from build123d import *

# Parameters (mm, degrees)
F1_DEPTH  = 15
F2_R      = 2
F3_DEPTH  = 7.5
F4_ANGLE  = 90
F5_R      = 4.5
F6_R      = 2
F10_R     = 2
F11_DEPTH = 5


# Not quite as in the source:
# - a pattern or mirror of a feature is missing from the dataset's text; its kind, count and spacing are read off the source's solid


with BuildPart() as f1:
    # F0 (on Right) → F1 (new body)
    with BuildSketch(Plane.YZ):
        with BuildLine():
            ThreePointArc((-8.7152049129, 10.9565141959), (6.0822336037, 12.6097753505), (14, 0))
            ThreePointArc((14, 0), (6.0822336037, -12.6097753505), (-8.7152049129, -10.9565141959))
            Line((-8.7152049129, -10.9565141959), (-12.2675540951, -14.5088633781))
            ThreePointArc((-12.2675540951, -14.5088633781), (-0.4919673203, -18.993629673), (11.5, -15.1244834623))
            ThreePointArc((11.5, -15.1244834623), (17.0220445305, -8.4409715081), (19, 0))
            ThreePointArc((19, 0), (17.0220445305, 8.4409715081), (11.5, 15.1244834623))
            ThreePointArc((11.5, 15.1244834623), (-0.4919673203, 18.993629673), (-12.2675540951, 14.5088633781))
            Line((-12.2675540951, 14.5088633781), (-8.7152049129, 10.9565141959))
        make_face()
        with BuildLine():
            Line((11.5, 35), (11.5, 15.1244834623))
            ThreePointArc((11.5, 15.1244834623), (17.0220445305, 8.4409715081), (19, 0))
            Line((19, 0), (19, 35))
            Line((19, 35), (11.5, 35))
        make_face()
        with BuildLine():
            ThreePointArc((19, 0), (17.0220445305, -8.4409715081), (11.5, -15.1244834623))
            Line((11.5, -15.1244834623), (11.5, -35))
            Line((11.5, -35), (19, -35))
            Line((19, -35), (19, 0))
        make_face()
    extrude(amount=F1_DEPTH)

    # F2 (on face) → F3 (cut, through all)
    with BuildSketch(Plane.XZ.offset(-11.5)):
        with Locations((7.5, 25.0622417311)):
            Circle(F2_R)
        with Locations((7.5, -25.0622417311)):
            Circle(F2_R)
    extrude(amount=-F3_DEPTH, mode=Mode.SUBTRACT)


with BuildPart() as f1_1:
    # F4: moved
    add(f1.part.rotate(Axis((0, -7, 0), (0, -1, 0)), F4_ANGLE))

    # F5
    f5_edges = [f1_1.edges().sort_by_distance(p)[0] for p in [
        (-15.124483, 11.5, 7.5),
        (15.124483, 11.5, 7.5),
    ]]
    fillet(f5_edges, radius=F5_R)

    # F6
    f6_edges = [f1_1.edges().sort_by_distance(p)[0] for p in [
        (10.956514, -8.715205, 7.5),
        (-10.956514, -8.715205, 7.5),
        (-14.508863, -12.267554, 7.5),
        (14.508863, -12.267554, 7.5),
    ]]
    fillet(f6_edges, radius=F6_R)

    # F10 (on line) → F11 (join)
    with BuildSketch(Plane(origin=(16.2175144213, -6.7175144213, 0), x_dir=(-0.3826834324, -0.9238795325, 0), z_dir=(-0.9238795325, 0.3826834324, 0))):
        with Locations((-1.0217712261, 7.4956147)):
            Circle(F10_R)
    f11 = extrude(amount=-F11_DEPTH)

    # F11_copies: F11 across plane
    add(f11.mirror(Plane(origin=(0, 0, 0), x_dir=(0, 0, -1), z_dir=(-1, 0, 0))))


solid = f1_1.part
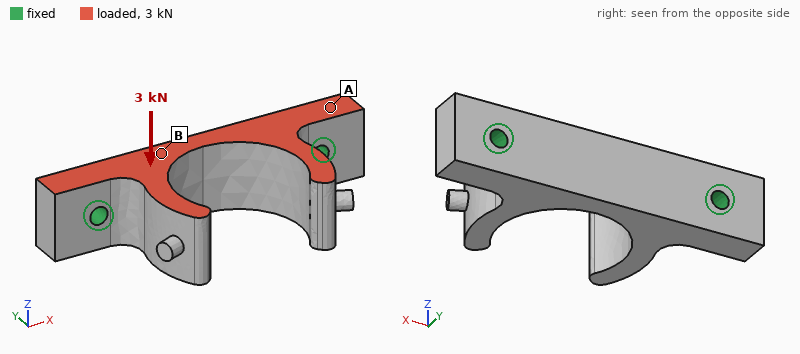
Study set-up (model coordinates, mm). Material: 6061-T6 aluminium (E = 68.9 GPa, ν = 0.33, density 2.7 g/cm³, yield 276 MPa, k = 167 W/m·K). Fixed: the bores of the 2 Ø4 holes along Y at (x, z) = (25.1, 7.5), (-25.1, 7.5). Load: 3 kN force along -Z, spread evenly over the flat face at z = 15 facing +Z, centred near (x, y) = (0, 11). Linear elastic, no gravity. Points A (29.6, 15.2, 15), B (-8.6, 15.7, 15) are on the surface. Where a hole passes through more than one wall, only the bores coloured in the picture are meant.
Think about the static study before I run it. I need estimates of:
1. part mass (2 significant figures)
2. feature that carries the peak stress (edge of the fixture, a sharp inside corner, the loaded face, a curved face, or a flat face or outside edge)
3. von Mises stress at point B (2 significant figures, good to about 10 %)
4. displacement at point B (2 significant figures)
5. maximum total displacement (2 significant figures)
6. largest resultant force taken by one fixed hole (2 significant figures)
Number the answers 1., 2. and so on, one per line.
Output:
1. 30 g
2. edge of the fixture
3. 19 MPa
4. 15 µm
5. 52 µm
6. 1.5 kN
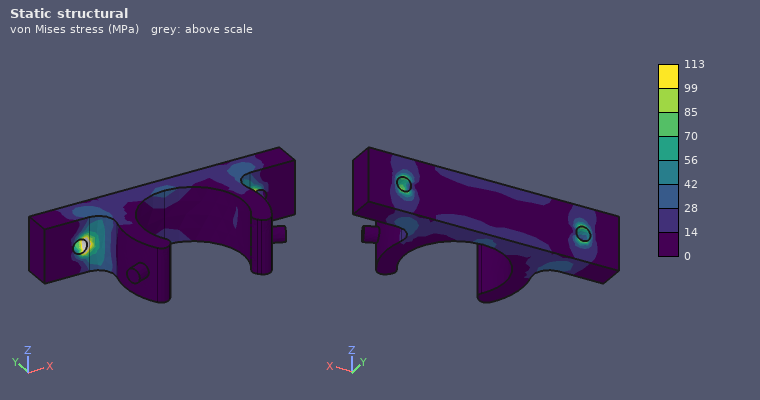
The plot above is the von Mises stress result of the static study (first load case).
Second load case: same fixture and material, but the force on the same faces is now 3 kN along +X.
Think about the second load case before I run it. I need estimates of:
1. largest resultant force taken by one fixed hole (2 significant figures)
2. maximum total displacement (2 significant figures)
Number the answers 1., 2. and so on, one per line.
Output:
1. 1.6 kN
2. 61 µm
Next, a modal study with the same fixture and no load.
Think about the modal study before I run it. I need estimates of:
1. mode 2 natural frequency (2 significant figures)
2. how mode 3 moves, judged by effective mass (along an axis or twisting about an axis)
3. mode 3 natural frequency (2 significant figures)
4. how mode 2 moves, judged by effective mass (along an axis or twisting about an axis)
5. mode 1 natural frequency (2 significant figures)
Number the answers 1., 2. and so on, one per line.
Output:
1. 8400 Hz
2. along X
3. 8900 Hz
4. along Z
5. 6800 Hz
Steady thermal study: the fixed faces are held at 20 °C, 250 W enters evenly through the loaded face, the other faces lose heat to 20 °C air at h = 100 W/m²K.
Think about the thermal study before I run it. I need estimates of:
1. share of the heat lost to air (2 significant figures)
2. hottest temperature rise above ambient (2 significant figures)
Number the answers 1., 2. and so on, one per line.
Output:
1. 6.9 %
2. 76 K
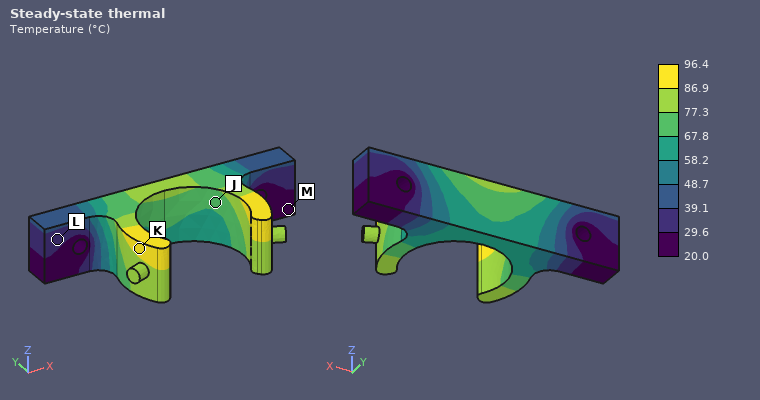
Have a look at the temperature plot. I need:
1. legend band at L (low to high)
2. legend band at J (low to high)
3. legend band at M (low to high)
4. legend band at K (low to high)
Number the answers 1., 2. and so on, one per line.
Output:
1. 29.6 to 39.1 °C
2. 67.8 to 77.3 °C
3. 20.0 to 29.6 °C
4. 86.9 to 96.4 °C
